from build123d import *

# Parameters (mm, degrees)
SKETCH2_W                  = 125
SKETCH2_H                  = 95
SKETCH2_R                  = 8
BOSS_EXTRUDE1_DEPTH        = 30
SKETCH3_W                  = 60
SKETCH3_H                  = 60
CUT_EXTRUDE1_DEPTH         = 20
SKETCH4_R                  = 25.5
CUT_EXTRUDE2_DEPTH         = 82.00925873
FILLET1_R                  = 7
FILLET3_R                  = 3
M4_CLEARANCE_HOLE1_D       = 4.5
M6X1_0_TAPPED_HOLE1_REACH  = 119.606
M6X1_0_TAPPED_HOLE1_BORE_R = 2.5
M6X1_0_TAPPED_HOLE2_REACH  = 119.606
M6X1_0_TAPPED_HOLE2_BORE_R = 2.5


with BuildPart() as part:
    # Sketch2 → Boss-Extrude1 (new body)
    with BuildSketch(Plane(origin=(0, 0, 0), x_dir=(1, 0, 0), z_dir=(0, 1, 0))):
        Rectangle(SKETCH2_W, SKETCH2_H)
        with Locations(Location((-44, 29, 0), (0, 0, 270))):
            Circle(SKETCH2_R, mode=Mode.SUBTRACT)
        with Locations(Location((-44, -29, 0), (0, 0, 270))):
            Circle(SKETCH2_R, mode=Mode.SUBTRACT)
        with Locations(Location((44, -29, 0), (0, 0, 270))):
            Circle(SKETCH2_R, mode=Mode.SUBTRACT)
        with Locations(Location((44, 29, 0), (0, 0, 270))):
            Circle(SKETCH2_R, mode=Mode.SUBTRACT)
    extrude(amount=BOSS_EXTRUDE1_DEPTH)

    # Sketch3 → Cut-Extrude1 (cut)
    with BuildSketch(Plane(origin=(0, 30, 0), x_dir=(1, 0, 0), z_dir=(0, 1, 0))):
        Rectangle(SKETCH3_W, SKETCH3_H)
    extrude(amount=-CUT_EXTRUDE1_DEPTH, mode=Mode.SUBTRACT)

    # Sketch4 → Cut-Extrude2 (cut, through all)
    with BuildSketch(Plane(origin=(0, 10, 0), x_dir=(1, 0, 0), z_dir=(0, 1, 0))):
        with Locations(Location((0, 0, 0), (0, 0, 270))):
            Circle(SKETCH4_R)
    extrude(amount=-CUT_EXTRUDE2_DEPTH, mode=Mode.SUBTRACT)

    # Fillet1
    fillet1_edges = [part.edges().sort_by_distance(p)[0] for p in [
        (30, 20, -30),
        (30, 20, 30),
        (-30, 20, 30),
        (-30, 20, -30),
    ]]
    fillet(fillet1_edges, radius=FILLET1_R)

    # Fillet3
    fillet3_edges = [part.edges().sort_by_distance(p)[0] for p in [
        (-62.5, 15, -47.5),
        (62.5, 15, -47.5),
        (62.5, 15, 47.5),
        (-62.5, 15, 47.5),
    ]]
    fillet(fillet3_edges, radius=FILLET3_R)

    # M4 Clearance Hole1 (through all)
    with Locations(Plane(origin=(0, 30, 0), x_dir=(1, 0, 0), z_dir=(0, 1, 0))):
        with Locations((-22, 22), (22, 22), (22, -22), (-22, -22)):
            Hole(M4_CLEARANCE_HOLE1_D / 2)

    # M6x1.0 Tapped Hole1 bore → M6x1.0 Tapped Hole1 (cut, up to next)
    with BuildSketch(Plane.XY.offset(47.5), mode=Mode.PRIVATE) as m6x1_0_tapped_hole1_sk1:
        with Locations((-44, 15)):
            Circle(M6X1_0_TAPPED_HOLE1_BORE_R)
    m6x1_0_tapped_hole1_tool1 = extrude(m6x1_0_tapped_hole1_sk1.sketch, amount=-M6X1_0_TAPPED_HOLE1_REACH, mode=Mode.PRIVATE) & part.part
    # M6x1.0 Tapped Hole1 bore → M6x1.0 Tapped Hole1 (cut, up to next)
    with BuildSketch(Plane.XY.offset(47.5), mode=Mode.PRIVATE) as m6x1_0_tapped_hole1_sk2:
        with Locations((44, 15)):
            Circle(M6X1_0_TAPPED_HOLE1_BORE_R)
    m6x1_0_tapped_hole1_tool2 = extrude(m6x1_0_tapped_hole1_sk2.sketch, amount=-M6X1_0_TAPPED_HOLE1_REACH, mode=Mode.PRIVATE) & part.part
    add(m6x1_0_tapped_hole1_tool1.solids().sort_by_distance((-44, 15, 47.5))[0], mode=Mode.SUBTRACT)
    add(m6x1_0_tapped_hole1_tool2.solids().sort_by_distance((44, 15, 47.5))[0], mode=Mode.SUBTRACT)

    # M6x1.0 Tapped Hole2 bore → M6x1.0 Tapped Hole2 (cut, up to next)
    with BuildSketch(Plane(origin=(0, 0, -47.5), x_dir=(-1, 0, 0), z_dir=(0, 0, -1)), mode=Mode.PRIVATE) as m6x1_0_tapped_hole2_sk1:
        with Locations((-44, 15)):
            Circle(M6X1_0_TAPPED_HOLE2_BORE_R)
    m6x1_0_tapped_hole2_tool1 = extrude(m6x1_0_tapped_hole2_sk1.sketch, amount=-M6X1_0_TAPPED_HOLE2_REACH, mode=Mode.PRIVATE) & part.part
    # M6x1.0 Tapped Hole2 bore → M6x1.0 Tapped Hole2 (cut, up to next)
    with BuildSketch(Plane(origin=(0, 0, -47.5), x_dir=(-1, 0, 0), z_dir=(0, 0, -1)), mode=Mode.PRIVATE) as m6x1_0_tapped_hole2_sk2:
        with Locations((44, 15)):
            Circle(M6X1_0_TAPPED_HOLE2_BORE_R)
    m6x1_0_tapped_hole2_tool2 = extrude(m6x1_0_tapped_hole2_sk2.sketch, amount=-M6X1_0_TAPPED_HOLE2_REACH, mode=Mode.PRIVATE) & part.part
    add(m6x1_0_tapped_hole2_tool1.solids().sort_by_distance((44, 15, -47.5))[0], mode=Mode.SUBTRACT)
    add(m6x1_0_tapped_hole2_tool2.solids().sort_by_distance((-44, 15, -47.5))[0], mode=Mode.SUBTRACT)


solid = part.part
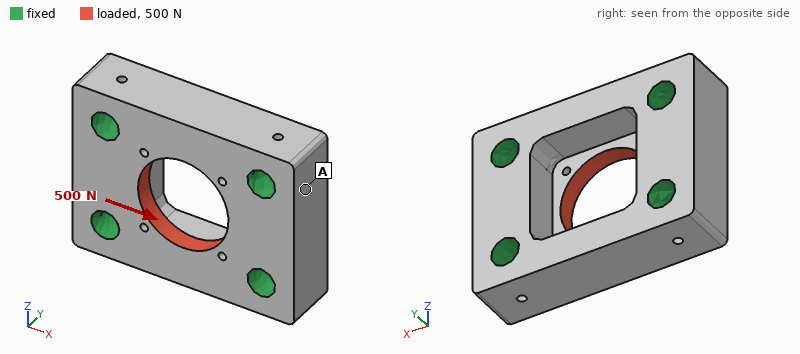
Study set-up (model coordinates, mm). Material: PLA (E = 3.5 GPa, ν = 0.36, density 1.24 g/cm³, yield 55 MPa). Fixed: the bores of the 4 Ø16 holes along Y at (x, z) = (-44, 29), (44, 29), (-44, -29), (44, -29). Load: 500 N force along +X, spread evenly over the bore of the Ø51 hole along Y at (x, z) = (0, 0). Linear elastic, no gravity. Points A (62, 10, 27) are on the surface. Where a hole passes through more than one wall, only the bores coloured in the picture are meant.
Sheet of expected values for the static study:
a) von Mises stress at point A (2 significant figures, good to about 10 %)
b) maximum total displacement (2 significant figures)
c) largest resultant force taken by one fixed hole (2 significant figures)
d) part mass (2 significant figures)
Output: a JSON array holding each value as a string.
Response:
["0.072 MPa", "3.5 µm", "130 N", "300 g"]
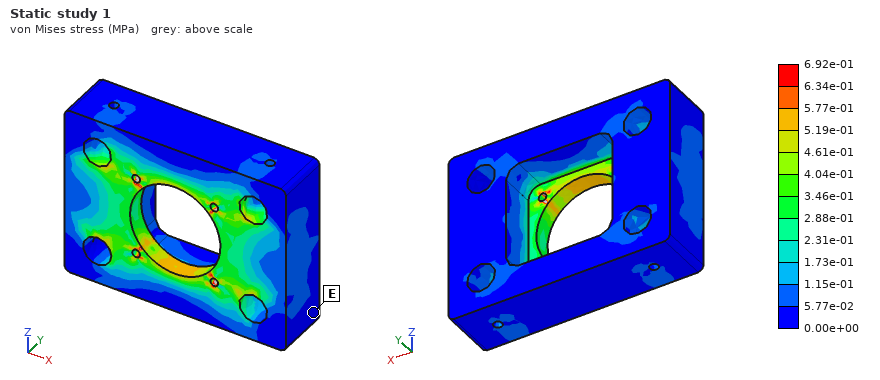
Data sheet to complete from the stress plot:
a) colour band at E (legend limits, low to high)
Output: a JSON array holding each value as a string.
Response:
["0.00e+00 to 5.77e-02 MPa"]
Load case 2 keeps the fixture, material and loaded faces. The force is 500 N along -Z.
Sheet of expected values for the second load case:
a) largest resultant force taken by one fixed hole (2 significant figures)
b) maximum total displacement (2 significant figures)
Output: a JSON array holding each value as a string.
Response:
["130 N", "8.7 µm"]
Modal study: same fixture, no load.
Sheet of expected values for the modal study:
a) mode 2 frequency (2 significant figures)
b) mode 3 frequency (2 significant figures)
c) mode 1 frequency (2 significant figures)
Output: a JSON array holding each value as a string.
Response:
["5000 Hz", "5100 Hz", "4900 Hz"]
